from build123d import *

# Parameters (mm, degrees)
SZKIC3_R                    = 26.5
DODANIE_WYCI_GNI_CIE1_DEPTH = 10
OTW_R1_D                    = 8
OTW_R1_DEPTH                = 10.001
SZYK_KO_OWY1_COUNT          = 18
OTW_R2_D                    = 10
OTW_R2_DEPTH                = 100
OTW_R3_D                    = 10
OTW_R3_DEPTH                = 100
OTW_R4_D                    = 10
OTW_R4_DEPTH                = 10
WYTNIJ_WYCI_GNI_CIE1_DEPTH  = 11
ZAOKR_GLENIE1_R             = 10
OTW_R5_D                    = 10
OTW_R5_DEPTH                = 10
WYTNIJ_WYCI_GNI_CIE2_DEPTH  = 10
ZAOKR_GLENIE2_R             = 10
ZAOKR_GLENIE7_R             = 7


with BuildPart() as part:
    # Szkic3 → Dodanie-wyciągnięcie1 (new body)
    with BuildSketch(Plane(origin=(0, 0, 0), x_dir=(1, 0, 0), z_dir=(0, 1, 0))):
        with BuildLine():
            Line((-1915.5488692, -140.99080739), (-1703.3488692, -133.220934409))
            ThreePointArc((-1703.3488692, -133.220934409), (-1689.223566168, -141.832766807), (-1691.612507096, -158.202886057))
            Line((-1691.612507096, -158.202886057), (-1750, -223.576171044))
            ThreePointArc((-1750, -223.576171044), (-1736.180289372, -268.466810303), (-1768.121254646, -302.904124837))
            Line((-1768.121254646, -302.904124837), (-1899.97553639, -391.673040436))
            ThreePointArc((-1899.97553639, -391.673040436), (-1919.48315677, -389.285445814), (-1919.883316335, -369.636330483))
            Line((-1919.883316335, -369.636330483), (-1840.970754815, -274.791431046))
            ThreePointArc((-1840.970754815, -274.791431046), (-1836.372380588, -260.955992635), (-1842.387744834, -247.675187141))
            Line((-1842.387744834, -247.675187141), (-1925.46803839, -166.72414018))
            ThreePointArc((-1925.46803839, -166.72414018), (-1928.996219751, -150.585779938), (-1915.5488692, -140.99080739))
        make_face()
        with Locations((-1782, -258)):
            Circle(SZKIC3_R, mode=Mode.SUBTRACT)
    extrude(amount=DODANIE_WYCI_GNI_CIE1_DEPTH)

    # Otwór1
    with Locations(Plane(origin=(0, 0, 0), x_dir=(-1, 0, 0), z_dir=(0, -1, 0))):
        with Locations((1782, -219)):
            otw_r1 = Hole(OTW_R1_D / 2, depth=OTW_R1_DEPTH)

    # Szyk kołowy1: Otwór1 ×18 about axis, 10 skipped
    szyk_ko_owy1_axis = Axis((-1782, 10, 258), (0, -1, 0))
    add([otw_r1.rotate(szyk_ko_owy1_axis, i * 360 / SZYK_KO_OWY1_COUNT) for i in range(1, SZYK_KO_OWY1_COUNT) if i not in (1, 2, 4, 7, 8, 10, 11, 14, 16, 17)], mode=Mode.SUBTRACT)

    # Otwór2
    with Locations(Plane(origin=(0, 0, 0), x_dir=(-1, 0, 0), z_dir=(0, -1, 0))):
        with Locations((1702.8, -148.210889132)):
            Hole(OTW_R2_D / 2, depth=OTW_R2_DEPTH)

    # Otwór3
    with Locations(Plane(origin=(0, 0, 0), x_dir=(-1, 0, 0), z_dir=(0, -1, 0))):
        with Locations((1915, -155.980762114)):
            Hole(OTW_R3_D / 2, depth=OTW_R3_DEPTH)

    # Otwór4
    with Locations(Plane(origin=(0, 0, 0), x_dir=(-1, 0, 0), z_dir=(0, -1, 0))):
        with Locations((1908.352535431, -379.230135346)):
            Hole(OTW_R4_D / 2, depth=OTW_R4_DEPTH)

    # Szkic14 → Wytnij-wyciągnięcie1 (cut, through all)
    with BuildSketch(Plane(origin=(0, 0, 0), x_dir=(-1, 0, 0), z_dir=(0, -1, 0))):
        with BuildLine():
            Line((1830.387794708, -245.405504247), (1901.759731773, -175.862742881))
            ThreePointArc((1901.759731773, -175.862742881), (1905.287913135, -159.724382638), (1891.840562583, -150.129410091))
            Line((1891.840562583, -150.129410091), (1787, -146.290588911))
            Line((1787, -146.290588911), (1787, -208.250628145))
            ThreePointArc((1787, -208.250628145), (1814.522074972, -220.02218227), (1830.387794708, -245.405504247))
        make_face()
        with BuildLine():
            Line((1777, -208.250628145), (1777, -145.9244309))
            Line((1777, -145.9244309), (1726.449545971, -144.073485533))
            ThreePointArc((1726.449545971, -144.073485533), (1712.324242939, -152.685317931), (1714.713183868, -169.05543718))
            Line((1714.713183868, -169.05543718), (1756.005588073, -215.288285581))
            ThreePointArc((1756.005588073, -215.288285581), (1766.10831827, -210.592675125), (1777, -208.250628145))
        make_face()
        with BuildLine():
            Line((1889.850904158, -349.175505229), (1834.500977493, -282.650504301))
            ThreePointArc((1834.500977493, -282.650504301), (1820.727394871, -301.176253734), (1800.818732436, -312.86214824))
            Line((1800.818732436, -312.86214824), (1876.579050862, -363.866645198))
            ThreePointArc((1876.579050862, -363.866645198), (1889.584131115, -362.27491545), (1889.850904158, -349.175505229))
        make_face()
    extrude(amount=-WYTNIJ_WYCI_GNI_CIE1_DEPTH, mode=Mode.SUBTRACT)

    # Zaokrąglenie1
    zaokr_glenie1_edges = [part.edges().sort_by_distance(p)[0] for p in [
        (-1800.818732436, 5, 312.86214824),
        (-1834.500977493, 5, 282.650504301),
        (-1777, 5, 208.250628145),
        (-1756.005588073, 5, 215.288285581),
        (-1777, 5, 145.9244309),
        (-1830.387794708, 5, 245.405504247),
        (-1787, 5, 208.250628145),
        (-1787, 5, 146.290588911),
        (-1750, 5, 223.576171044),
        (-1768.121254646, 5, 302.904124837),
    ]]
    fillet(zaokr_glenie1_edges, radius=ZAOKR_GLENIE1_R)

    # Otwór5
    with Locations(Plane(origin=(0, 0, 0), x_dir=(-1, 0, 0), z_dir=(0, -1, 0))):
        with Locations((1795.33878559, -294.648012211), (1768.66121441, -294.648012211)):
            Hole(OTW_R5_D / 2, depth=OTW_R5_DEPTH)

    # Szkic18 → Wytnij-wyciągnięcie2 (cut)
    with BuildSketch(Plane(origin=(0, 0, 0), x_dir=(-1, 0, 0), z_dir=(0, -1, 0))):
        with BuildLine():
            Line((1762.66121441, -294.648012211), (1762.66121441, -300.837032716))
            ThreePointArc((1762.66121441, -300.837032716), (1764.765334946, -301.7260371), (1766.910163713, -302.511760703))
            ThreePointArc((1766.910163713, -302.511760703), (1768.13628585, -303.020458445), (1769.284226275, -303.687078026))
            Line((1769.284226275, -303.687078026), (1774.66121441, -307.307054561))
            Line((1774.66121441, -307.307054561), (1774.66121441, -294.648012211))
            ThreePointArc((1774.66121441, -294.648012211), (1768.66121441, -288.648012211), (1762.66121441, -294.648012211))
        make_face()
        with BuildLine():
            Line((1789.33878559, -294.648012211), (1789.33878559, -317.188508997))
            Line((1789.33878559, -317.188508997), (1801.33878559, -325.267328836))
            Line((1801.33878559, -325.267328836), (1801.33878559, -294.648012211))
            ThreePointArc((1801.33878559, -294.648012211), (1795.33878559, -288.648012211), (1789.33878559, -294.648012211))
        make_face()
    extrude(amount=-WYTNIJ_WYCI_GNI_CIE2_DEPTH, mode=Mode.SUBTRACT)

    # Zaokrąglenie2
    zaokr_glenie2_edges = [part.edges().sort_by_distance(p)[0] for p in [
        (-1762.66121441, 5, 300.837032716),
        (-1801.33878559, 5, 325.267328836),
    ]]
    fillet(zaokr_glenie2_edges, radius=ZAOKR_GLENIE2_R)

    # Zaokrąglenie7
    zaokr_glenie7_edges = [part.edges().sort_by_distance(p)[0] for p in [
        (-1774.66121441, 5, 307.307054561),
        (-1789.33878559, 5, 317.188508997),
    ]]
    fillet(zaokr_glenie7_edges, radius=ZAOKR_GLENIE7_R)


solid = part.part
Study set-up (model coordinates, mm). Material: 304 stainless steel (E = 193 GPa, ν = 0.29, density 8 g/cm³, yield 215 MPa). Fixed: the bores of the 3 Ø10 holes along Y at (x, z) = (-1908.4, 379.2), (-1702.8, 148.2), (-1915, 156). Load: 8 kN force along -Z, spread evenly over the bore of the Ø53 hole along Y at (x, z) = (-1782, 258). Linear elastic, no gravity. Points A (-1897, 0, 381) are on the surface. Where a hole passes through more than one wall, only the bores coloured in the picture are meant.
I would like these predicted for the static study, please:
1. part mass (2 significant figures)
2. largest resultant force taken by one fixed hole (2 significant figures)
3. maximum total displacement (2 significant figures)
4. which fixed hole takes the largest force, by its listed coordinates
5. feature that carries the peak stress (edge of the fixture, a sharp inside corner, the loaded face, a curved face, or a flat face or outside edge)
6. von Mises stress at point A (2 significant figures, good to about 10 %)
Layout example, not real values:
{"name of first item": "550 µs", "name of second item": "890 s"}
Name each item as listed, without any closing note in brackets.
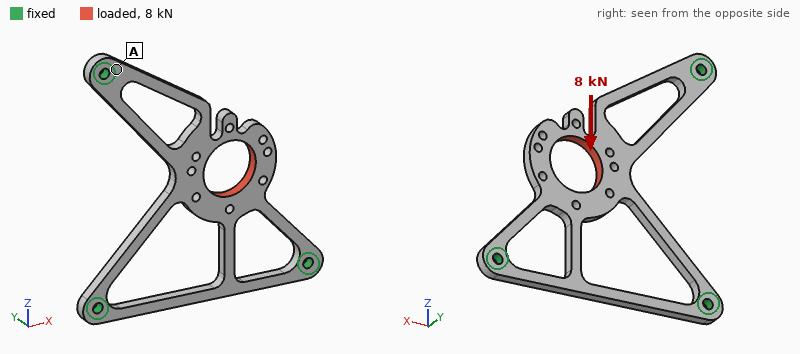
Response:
{"part mass": "1.1 kg", "largest resultant force taken by one fixed hole": "4.7 kN", "maximum total displacement": "0.11 mm", "which fixed hole takes the largest force, by its listed coordinates": "(-1915, 156)", "feature that carries the peak stress": "a curved face", "von Mises stress at point A": "13 MPa"}
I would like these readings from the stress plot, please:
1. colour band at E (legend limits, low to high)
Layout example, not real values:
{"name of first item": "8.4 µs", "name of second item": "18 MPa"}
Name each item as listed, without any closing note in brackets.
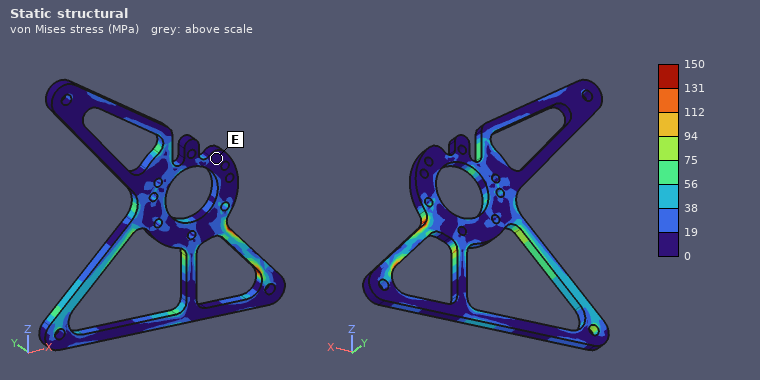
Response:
{"colour band at E": "0 to 19 MPa"}
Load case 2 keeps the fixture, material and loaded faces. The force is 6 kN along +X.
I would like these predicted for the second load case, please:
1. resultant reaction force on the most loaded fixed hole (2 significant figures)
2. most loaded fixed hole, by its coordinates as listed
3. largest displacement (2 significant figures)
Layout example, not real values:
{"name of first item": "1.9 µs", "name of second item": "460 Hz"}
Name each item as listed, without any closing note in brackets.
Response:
{"resultant reaction force on the most loaded fixed hole": "4.0 kN", "most loaded fixed hole, by its coordinates as listed": "(-1915, 156)", "largest displacement": "63 µm"}
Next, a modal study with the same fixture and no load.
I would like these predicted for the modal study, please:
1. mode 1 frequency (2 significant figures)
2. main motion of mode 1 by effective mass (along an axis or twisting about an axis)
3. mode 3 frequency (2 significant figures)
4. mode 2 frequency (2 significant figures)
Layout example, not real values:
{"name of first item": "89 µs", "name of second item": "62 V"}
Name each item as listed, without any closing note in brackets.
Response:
{"mode 1 frequency": "400 Hz", "main motion of mode 1 by effective mass": "along Y", "mode 3 frequency": "1200 Hz", "mode 2 frequency": "950 Hz"}
